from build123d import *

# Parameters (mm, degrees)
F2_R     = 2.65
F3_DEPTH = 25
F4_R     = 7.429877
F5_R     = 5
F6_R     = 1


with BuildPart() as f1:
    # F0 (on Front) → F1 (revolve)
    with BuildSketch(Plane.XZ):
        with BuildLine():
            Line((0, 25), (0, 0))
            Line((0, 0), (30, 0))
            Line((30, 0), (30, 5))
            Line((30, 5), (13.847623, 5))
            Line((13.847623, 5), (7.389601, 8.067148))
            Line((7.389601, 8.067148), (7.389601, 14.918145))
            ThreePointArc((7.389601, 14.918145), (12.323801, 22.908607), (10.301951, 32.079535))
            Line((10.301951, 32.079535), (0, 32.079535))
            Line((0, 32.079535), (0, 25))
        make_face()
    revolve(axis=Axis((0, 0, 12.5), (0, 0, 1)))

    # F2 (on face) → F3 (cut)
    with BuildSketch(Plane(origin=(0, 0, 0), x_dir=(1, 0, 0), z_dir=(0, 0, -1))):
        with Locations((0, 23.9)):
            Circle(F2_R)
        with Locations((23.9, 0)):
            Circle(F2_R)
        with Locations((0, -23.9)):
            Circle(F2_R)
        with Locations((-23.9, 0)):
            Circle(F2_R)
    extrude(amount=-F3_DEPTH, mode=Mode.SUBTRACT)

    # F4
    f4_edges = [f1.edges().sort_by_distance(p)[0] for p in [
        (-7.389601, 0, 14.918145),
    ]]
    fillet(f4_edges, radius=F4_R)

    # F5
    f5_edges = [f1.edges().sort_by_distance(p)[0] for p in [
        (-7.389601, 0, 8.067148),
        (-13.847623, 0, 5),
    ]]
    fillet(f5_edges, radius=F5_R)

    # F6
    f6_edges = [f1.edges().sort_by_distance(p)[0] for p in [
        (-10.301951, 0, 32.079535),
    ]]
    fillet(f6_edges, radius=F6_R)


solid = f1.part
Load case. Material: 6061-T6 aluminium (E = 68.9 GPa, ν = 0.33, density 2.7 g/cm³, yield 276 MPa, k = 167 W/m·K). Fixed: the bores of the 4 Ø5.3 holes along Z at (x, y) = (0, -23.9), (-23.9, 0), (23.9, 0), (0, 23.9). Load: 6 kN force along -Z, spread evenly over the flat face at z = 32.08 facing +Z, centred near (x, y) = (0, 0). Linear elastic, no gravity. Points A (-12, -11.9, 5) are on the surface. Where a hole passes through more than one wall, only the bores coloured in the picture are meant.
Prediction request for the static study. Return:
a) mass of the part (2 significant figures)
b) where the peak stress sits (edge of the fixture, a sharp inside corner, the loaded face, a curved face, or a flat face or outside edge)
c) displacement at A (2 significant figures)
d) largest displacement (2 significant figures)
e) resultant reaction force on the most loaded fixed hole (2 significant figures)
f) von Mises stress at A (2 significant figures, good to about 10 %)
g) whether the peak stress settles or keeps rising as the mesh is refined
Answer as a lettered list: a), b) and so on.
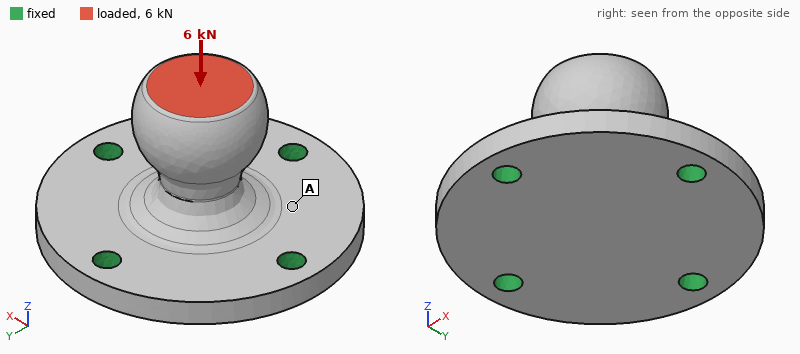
a) 62 g
b) edge of the fixture
c) 20 µm
d) 45 µm
e) 1.6 kN
f) 33 MPa
g) keeps rising
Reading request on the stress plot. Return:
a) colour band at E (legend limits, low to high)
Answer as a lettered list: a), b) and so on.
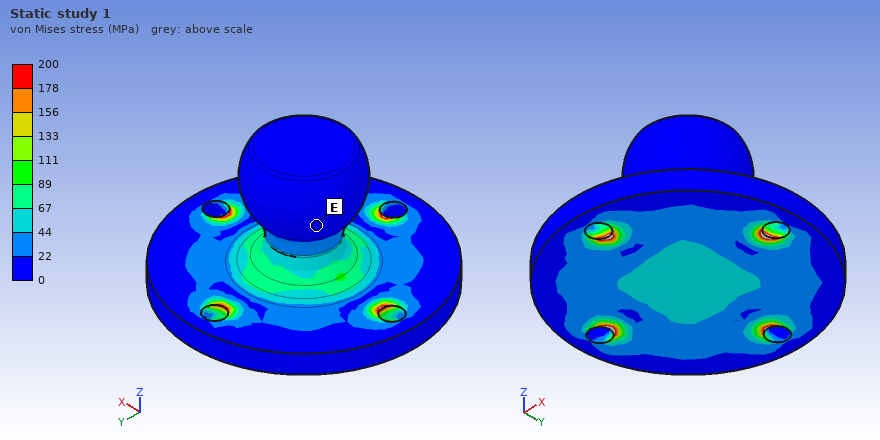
a) 0 to 22 MPa
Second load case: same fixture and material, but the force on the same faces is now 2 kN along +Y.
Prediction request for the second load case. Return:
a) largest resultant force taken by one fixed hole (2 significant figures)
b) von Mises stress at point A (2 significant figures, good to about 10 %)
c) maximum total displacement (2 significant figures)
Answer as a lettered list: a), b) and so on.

a) 1.6 kN
b) 31 MPa
c) 0.13 mm
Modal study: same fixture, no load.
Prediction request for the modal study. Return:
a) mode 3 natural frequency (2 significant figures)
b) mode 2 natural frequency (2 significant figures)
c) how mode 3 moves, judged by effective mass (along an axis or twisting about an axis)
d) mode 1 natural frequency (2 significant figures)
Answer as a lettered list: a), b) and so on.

a) 11 kHz
b) 6300 Hz
c) along Z
d) 6300 Hz
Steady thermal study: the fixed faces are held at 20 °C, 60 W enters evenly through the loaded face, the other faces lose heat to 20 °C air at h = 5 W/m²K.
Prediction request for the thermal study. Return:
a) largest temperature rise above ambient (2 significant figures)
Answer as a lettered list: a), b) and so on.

a) 52 K
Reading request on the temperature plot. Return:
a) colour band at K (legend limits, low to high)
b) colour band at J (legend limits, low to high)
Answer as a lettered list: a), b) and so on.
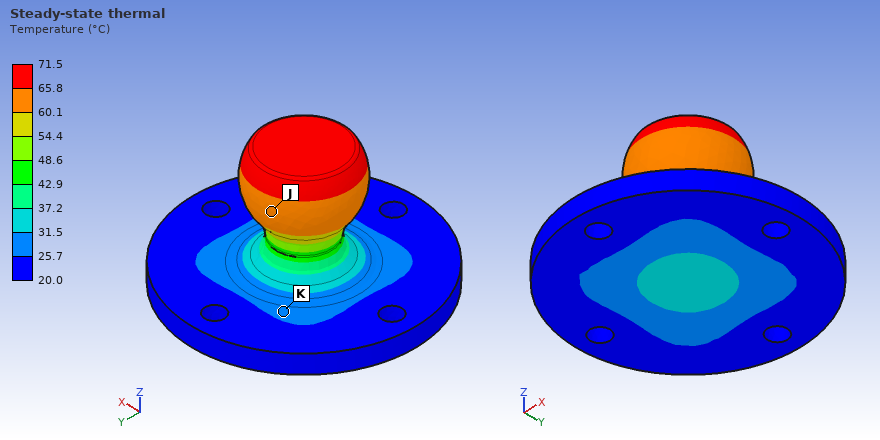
a) 25.7 to 31.5 °C
b) 60.1 to 65.8 °C
